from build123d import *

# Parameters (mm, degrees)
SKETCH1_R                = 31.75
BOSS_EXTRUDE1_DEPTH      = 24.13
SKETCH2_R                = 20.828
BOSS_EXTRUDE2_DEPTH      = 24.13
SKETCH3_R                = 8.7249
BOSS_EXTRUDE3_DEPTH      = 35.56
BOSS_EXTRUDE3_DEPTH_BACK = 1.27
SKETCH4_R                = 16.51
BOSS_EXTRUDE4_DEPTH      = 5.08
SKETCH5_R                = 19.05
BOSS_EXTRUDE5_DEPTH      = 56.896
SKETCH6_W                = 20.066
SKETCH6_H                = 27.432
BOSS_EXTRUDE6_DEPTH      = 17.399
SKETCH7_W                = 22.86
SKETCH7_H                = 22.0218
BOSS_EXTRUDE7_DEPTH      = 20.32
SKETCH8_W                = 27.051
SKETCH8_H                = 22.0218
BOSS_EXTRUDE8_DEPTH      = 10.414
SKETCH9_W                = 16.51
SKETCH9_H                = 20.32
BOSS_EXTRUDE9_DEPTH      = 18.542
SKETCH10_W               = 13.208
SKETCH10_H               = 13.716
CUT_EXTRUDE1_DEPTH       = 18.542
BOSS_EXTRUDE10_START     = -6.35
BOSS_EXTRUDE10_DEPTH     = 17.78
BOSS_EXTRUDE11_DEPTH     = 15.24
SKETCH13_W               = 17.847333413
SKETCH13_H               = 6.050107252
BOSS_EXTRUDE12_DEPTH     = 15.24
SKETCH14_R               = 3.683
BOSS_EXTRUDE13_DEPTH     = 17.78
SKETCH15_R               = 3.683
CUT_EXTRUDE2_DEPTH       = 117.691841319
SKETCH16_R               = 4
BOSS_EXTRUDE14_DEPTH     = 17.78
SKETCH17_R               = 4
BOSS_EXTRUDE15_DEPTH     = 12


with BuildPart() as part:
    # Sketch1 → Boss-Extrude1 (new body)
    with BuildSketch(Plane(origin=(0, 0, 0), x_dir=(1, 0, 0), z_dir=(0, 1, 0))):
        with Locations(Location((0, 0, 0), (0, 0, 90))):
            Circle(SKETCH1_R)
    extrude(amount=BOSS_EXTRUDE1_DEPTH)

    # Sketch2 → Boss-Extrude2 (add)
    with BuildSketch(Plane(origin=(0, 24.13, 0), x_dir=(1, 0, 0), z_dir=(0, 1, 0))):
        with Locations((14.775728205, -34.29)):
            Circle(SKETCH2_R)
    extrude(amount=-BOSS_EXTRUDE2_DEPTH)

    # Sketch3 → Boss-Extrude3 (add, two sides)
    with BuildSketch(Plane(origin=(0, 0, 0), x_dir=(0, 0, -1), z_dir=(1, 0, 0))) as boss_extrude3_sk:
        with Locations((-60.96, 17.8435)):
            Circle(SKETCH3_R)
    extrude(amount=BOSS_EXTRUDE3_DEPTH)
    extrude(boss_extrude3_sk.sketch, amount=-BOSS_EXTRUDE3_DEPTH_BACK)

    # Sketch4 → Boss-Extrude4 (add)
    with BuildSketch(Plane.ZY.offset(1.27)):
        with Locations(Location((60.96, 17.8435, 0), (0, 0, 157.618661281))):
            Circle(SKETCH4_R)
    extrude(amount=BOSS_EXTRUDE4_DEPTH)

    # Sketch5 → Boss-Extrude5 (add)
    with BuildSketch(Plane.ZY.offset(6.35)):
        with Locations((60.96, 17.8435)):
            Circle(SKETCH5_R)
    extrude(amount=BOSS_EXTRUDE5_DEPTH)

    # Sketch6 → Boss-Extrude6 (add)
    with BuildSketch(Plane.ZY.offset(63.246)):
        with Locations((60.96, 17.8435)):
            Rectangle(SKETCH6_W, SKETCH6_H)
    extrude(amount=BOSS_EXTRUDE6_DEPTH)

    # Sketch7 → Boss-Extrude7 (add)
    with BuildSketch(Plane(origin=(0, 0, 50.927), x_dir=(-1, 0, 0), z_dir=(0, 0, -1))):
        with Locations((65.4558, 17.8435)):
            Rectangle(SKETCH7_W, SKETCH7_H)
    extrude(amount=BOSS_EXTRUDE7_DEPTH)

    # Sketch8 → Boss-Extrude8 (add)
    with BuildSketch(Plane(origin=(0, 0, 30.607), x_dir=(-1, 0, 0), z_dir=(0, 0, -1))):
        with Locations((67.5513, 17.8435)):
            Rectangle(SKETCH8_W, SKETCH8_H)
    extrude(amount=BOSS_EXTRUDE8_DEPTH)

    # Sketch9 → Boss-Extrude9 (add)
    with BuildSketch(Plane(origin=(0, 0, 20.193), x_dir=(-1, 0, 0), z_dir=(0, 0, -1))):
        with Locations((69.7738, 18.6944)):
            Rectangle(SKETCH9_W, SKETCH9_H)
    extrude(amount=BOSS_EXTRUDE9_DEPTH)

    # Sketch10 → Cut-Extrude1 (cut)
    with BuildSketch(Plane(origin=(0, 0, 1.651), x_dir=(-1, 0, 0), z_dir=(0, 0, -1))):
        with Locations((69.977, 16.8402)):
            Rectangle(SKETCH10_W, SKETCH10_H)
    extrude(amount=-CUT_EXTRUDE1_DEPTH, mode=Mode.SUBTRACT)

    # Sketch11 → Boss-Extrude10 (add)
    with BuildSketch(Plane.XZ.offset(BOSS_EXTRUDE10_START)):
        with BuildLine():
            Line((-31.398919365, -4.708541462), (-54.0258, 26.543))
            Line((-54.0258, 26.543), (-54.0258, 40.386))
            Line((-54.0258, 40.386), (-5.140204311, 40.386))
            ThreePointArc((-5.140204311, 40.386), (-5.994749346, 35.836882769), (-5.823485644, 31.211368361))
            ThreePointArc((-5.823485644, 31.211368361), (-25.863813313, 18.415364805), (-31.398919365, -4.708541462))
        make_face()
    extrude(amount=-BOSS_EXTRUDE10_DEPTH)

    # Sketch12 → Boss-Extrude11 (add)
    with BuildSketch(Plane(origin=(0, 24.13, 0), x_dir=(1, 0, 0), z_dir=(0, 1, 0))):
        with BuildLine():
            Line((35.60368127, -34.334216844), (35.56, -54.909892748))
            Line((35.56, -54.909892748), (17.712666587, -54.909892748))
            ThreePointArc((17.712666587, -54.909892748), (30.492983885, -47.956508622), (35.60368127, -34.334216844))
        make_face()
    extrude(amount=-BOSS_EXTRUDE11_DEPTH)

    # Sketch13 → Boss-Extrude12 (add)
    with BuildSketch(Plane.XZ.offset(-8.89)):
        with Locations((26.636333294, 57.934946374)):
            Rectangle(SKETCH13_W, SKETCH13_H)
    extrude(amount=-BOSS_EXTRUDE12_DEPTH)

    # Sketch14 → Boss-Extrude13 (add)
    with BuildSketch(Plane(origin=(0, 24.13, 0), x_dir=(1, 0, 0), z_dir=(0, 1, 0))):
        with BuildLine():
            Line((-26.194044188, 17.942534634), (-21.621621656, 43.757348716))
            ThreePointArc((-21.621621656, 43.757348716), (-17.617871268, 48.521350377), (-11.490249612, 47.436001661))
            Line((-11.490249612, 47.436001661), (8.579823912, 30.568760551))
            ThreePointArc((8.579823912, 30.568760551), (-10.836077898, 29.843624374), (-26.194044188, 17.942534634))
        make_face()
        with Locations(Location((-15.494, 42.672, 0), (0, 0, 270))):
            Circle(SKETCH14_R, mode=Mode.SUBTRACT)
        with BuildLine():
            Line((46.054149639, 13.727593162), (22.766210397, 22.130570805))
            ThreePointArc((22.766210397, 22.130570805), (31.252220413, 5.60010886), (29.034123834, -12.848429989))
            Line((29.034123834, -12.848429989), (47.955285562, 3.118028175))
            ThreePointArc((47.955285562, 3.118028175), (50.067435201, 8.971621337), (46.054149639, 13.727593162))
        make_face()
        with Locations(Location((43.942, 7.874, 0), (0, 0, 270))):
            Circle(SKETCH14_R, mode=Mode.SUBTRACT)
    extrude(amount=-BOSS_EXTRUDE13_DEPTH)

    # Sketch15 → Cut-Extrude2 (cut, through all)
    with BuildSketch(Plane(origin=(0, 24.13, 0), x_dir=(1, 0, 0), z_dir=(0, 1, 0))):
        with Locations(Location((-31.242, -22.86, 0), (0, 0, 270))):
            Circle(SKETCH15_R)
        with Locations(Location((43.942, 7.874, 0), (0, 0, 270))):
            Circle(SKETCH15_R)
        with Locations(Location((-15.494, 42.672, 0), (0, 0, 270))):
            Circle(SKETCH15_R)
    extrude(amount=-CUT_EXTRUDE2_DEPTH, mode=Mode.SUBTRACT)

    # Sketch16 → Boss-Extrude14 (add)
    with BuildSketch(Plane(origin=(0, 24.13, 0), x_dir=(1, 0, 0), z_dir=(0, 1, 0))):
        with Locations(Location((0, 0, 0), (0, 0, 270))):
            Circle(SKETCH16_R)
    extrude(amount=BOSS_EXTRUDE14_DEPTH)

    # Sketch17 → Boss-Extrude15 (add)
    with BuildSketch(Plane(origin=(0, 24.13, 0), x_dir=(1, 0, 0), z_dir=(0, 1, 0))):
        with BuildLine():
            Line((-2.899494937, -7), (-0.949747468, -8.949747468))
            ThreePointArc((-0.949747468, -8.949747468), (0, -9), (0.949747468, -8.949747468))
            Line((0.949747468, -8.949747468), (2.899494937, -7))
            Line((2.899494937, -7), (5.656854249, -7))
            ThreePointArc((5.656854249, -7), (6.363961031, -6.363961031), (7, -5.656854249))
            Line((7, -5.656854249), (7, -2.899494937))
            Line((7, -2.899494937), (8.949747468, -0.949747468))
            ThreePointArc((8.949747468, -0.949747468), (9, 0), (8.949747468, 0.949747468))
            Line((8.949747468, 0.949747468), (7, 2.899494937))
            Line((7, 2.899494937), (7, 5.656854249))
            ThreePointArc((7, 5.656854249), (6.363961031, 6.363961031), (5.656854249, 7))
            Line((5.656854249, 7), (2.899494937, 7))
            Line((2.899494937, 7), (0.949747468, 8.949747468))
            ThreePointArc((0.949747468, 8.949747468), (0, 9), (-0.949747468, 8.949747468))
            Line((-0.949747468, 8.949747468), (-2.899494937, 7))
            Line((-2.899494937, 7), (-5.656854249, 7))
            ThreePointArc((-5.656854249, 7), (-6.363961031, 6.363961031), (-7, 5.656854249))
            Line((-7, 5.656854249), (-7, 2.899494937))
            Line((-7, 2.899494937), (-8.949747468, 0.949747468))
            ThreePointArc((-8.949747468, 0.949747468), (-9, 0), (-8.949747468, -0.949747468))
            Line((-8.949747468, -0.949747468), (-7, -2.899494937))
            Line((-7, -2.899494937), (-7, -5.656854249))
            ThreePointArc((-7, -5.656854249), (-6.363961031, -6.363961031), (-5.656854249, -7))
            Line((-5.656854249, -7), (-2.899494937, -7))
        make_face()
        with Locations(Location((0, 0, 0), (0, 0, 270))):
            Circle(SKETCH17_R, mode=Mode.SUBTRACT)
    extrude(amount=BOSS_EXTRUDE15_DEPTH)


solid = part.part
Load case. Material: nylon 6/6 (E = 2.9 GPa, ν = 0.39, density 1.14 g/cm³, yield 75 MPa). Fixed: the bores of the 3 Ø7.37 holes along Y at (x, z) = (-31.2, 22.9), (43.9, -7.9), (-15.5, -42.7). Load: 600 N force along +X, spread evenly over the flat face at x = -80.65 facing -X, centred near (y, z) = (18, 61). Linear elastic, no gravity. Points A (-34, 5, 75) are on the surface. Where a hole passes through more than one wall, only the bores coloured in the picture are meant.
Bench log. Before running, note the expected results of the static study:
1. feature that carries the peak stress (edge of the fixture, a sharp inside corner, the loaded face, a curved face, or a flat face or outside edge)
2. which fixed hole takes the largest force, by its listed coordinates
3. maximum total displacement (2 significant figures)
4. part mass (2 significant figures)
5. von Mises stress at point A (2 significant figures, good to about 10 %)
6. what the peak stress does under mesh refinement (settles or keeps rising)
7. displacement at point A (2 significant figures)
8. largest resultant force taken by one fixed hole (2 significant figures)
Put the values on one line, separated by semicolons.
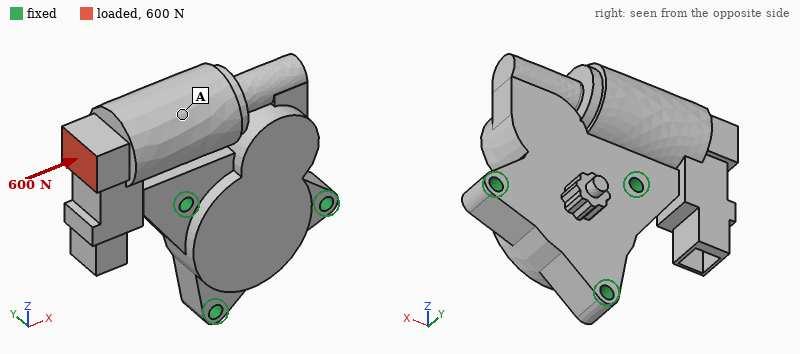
edge of the fixture; (-31.2, 22.9); 0.12 mm; 270 g; 0.60 MPa; keeps rising; 0.076 mm; 680 N
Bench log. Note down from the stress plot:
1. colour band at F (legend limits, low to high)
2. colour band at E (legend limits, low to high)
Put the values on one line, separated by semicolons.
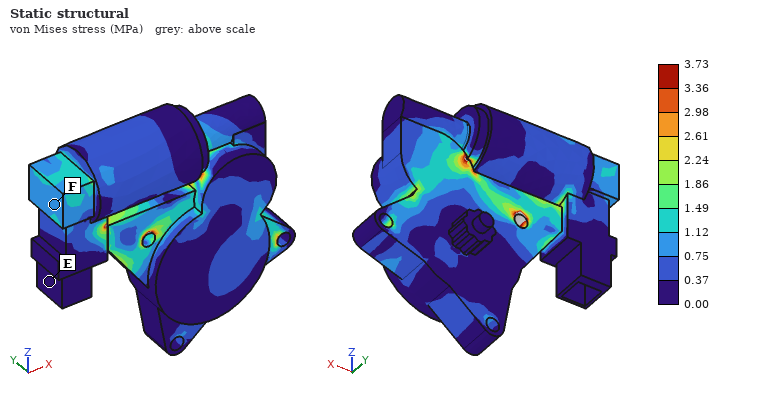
0.75 to 1.12 MPa; 0.00 to 0.37 MPa
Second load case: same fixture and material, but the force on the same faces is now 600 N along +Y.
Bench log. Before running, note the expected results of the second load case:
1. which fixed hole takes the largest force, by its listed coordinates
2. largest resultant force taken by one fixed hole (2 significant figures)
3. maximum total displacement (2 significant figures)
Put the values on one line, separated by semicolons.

(-31.2, 22.9); 880 N; 1.1 mm
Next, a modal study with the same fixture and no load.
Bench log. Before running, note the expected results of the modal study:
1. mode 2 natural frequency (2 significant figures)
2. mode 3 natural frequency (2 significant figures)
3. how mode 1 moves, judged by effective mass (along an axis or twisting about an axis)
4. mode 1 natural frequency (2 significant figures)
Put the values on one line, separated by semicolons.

1000 Hz; 1200 Hz; along Y; 600 Hz
